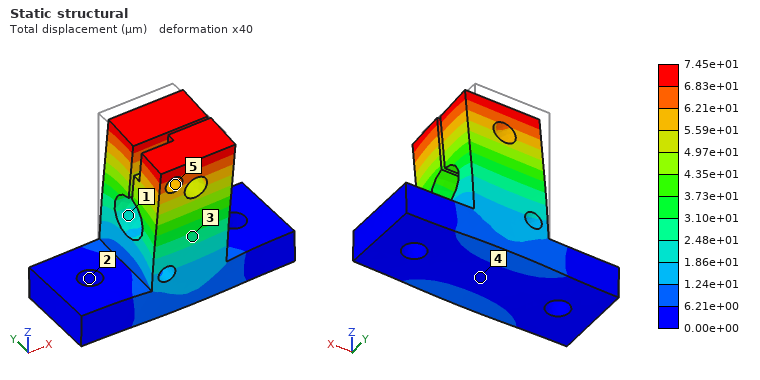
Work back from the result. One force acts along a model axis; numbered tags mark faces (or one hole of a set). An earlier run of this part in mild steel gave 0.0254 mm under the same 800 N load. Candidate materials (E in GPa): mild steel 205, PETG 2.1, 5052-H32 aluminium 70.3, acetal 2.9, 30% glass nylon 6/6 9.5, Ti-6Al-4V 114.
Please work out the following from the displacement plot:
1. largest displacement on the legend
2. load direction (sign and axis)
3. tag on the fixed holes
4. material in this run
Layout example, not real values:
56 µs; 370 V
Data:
7.45e+01 µm; -Y; 2; 5052-H32 aluminium
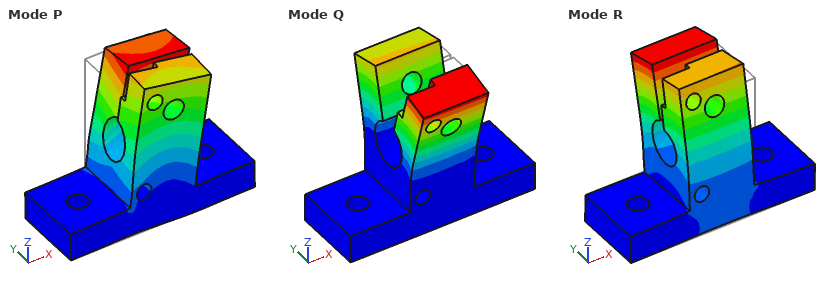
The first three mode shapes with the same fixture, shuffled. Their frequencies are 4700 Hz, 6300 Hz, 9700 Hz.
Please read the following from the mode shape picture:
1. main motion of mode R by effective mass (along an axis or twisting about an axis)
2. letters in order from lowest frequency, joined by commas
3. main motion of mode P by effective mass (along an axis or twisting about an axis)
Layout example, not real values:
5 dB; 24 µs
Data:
along Y; R, Q, P; along X
